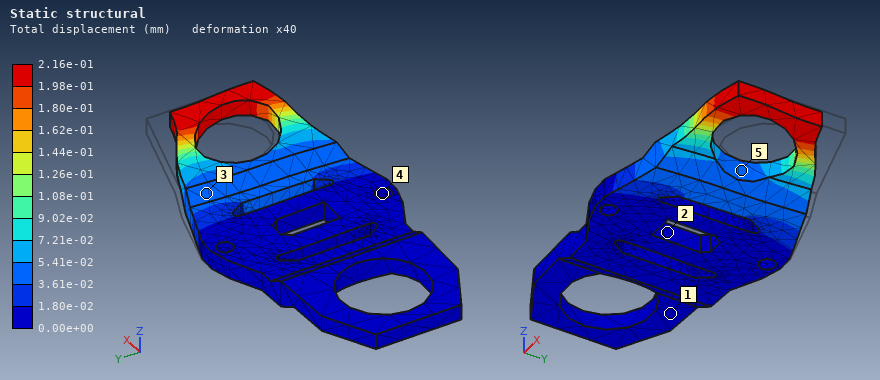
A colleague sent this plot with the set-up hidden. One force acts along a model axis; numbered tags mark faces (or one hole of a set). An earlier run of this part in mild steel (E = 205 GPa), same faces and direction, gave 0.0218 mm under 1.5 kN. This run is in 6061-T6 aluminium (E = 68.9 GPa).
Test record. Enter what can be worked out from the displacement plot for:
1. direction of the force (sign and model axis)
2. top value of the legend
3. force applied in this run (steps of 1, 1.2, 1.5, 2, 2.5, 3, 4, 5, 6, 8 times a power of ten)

-Y
2.16e-01 mm
5 kN
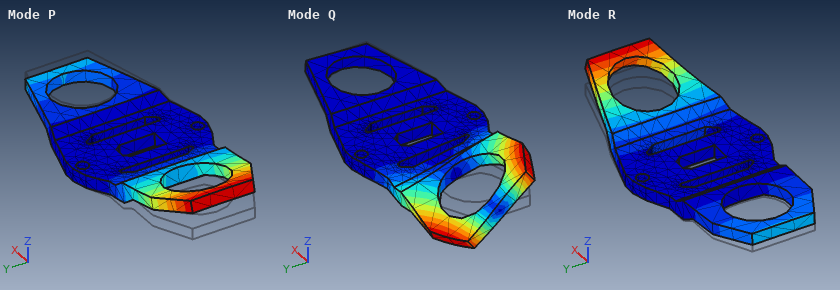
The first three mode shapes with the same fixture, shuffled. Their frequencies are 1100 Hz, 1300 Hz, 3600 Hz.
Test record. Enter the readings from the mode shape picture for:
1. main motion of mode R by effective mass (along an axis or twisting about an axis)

along Z
